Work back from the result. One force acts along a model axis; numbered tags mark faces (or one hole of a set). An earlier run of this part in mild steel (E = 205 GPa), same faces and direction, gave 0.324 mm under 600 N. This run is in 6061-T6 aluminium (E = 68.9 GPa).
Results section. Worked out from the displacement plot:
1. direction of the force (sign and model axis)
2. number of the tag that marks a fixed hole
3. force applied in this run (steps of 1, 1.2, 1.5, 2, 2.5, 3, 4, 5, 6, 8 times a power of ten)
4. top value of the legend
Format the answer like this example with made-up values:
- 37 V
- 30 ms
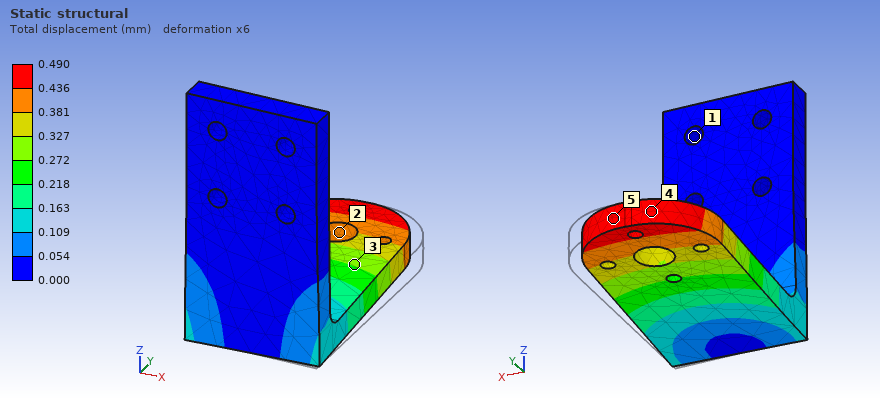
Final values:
- -X
- 1
- 300 N
- 0.490 mm
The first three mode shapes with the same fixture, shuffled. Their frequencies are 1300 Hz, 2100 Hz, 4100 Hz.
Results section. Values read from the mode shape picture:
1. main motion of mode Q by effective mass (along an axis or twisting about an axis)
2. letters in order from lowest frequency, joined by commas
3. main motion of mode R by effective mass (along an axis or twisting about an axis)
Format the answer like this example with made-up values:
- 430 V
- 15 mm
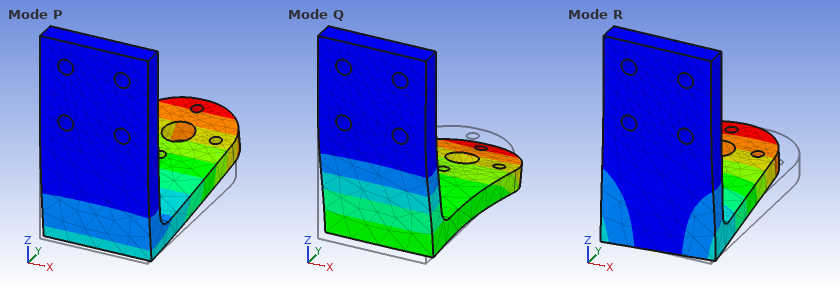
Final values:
- along Y
- P, R, Q
- along X
